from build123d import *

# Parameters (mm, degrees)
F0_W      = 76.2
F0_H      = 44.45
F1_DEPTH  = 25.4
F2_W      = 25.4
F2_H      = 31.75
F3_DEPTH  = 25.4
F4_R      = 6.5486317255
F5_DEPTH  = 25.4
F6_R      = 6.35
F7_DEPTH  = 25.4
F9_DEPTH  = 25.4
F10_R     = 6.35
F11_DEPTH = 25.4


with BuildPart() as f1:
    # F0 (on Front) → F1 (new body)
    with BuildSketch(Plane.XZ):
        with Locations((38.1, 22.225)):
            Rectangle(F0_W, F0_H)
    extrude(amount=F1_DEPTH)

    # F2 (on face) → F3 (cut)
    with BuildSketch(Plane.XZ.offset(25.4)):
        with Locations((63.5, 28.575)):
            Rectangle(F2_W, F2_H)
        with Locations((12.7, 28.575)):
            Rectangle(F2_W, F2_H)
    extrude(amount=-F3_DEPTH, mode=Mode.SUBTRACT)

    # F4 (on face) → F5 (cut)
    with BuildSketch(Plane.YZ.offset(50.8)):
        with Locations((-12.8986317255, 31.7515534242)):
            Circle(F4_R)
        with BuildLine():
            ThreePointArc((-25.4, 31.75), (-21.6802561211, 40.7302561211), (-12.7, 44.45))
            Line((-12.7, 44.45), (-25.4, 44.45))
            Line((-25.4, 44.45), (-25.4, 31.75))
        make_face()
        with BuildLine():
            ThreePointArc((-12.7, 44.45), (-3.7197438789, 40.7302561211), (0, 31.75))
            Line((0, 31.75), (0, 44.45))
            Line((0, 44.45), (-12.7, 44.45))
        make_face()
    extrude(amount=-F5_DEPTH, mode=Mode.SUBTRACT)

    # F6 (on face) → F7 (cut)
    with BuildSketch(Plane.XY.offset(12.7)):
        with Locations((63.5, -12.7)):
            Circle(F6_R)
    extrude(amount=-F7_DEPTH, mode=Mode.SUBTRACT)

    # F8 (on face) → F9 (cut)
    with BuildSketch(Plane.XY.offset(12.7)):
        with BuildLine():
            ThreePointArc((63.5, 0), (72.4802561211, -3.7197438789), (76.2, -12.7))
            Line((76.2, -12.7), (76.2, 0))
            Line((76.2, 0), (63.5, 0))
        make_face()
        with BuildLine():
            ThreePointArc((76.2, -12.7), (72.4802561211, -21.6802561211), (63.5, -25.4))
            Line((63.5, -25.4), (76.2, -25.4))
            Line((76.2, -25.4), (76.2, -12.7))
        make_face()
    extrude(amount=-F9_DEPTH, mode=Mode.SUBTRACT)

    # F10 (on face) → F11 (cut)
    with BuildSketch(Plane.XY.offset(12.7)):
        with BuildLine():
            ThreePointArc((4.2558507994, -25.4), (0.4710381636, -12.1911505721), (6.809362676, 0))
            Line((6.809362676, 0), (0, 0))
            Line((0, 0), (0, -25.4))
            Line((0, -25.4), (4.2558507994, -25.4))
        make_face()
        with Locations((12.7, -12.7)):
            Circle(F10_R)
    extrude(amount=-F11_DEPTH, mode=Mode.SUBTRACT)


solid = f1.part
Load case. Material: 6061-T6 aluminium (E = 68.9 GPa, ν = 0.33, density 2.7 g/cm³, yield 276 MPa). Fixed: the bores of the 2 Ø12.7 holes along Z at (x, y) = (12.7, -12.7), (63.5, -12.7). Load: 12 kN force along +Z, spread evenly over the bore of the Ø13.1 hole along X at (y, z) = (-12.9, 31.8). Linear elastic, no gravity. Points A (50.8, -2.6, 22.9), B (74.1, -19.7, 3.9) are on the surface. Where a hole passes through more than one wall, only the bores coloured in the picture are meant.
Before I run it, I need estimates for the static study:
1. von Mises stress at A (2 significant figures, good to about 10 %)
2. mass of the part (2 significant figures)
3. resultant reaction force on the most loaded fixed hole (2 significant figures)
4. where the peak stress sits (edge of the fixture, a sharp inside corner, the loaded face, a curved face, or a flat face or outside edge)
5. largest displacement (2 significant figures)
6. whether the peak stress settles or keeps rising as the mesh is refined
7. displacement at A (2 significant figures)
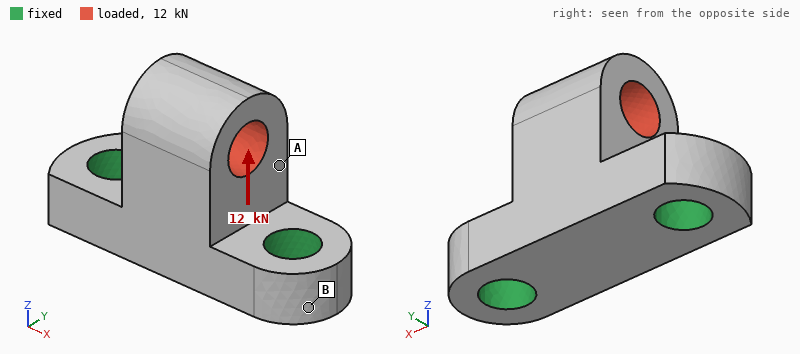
22 MPa
95 g
6.3 kN
edge of the fixture
28 µm
keeps rising
17 µm
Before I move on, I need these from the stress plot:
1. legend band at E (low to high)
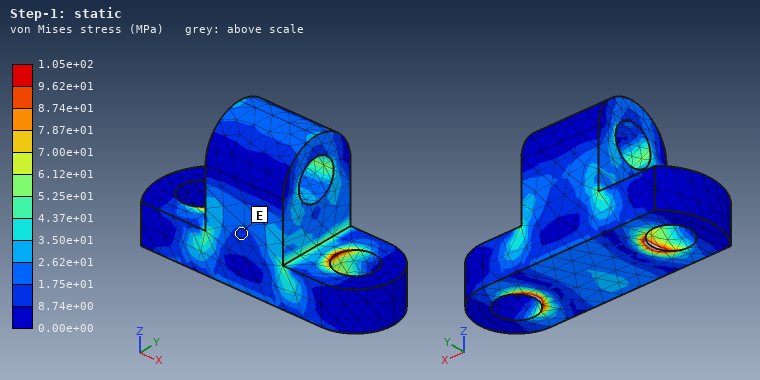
8.74e+00 to 1.75e+01 MPa
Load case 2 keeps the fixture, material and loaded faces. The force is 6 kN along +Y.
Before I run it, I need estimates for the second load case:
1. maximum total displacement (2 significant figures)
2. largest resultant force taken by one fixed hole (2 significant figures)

0.13 mm
3.0 kN
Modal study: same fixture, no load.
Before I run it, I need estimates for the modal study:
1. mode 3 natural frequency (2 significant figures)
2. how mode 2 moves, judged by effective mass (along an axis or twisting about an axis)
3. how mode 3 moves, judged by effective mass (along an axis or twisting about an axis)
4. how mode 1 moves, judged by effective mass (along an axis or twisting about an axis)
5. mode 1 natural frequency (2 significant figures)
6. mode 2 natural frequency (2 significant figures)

17 kHz
along X
along Z
along Y
7000 Hz
12 kHz
